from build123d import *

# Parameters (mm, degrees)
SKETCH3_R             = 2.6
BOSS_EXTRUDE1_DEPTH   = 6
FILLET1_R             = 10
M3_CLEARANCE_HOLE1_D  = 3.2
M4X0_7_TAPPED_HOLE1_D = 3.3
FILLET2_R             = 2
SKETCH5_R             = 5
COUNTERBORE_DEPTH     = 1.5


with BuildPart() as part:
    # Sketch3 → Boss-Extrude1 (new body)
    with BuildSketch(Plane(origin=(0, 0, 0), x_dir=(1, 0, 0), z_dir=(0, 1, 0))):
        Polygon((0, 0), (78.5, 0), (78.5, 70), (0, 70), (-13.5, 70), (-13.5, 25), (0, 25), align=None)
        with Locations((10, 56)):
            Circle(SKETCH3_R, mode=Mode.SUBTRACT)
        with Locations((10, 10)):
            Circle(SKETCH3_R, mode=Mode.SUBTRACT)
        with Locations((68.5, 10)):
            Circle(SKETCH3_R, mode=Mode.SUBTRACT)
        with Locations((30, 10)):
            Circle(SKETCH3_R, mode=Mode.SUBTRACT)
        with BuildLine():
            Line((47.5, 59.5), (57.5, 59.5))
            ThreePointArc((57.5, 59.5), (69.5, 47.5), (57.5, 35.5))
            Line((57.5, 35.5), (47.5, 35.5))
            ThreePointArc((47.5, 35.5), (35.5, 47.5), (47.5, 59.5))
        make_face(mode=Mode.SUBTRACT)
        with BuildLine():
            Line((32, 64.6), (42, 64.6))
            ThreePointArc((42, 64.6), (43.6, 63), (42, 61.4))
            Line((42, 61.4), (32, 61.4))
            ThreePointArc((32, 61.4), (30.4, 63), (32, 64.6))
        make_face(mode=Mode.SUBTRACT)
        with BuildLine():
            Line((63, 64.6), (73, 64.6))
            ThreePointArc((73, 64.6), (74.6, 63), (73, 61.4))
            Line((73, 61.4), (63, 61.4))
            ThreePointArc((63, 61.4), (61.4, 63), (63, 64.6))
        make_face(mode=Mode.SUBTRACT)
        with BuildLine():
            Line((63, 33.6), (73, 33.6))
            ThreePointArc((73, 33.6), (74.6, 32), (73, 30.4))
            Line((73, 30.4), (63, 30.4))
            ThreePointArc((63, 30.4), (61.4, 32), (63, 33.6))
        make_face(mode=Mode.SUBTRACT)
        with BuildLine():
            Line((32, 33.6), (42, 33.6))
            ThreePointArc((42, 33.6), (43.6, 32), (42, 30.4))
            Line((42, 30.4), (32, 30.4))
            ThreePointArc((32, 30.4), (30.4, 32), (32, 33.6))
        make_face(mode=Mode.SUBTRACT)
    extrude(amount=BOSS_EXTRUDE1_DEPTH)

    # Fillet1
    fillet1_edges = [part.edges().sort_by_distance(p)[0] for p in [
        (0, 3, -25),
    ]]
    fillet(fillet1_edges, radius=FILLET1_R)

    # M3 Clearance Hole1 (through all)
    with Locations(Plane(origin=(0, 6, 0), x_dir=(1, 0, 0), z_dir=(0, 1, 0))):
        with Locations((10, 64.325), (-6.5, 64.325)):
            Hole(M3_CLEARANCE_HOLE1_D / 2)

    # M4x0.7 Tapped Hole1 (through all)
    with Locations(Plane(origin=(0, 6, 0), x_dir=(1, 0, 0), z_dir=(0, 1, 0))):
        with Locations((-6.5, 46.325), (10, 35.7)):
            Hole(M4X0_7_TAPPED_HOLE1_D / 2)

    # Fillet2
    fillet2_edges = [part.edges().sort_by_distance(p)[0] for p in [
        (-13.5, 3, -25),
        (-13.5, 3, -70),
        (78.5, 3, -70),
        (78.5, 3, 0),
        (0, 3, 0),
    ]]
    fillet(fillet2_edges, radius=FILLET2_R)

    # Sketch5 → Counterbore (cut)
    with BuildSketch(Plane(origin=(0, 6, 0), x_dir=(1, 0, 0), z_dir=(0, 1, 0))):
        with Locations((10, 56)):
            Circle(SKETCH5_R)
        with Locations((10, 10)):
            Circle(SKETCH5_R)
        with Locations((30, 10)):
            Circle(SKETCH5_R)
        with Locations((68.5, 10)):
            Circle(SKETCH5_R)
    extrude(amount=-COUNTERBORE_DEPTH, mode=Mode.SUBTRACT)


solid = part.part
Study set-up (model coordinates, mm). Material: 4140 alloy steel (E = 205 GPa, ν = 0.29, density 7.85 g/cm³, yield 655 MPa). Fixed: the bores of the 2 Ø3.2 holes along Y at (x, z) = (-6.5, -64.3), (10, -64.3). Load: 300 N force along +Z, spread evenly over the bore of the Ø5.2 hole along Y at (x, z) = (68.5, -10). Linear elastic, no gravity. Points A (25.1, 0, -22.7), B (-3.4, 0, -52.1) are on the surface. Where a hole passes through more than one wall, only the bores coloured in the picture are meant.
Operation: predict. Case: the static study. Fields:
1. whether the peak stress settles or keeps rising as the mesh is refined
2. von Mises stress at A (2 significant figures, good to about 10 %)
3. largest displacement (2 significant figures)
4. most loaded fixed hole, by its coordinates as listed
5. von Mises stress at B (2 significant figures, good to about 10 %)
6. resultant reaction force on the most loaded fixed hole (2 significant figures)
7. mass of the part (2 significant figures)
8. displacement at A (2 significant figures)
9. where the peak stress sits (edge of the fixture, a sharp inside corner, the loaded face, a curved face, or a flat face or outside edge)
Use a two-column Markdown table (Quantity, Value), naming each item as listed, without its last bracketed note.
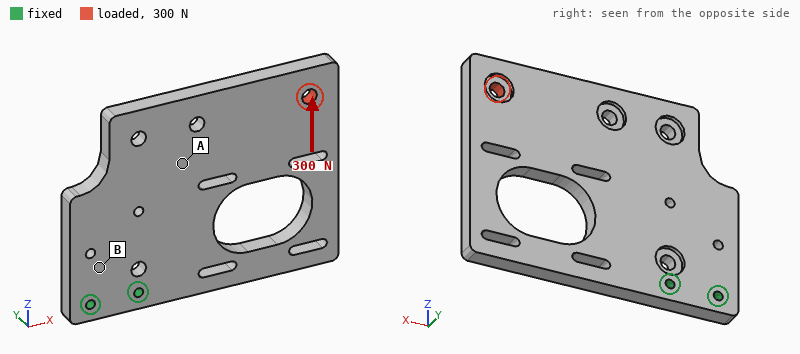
| Quantity | Value |
|---|---|
| whether the peak stress settles or keeps rising as the mesh is refined | keeps rising |
| von Mises stress at A | 3.6 MPa |
| largest displacement | 20 µm |
| most loaded fixed hole, by its coordinates as listed | (10, -64.3) |
| von Mises stress at B | 9.4 MPa |
| resultant reaction force on the most loaded fixed hole | 1.2 kN |
| mass of the part | 240 g |
| displacement at A | 7.5 µm |
| where the peak stress sits | edge of the fixture |
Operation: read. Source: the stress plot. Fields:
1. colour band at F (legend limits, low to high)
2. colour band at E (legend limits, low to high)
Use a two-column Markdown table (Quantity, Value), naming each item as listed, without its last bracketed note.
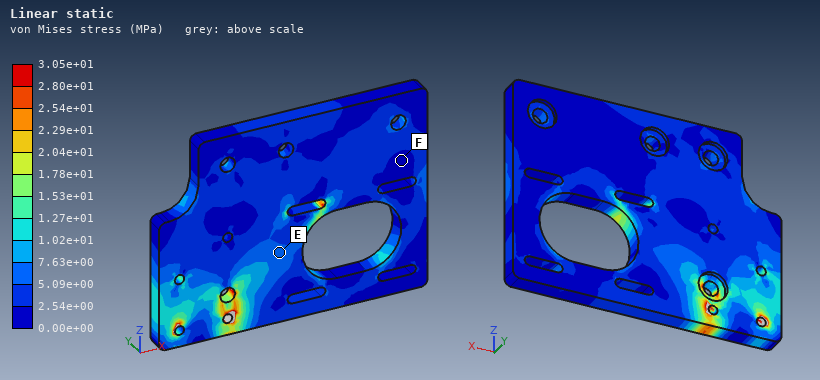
| Quantity | Value |
|---|---|
| colour band at F | 0.00e+00 to 2.54e+00 MPa |
| colour band at E | 5.09e+00 to 7.63e+00 MPa |
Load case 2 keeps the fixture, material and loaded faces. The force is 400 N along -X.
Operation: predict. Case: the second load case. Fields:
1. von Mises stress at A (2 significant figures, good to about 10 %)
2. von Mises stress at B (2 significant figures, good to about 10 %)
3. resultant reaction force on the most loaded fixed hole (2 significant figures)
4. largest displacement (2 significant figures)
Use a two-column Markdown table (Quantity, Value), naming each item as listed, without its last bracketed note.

| Quantity | Value |
|---|---|
| von Mises stress at A | 4.6 MPa |
| von Mises stress at B | 13 MPa |
| resultant reaction force on the most loaded fixed hole | 1.2 kN |
| largest displacement | 20 µm |
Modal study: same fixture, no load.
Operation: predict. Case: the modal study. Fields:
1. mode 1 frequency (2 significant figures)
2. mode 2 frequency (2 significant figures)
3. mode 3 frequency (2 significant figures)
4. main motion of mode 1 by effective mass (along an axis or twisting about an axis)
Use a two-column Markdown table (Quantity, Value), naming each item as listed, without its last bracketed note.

| Quantity | Value |
|---|---|
| mode 1 frequency | 570 Hz |
| mode 2 frequency | 1200 Hz |
| mode 3 frequency | 2100 Hz |
| main motion of mode 1 by effective mass | along Y |
